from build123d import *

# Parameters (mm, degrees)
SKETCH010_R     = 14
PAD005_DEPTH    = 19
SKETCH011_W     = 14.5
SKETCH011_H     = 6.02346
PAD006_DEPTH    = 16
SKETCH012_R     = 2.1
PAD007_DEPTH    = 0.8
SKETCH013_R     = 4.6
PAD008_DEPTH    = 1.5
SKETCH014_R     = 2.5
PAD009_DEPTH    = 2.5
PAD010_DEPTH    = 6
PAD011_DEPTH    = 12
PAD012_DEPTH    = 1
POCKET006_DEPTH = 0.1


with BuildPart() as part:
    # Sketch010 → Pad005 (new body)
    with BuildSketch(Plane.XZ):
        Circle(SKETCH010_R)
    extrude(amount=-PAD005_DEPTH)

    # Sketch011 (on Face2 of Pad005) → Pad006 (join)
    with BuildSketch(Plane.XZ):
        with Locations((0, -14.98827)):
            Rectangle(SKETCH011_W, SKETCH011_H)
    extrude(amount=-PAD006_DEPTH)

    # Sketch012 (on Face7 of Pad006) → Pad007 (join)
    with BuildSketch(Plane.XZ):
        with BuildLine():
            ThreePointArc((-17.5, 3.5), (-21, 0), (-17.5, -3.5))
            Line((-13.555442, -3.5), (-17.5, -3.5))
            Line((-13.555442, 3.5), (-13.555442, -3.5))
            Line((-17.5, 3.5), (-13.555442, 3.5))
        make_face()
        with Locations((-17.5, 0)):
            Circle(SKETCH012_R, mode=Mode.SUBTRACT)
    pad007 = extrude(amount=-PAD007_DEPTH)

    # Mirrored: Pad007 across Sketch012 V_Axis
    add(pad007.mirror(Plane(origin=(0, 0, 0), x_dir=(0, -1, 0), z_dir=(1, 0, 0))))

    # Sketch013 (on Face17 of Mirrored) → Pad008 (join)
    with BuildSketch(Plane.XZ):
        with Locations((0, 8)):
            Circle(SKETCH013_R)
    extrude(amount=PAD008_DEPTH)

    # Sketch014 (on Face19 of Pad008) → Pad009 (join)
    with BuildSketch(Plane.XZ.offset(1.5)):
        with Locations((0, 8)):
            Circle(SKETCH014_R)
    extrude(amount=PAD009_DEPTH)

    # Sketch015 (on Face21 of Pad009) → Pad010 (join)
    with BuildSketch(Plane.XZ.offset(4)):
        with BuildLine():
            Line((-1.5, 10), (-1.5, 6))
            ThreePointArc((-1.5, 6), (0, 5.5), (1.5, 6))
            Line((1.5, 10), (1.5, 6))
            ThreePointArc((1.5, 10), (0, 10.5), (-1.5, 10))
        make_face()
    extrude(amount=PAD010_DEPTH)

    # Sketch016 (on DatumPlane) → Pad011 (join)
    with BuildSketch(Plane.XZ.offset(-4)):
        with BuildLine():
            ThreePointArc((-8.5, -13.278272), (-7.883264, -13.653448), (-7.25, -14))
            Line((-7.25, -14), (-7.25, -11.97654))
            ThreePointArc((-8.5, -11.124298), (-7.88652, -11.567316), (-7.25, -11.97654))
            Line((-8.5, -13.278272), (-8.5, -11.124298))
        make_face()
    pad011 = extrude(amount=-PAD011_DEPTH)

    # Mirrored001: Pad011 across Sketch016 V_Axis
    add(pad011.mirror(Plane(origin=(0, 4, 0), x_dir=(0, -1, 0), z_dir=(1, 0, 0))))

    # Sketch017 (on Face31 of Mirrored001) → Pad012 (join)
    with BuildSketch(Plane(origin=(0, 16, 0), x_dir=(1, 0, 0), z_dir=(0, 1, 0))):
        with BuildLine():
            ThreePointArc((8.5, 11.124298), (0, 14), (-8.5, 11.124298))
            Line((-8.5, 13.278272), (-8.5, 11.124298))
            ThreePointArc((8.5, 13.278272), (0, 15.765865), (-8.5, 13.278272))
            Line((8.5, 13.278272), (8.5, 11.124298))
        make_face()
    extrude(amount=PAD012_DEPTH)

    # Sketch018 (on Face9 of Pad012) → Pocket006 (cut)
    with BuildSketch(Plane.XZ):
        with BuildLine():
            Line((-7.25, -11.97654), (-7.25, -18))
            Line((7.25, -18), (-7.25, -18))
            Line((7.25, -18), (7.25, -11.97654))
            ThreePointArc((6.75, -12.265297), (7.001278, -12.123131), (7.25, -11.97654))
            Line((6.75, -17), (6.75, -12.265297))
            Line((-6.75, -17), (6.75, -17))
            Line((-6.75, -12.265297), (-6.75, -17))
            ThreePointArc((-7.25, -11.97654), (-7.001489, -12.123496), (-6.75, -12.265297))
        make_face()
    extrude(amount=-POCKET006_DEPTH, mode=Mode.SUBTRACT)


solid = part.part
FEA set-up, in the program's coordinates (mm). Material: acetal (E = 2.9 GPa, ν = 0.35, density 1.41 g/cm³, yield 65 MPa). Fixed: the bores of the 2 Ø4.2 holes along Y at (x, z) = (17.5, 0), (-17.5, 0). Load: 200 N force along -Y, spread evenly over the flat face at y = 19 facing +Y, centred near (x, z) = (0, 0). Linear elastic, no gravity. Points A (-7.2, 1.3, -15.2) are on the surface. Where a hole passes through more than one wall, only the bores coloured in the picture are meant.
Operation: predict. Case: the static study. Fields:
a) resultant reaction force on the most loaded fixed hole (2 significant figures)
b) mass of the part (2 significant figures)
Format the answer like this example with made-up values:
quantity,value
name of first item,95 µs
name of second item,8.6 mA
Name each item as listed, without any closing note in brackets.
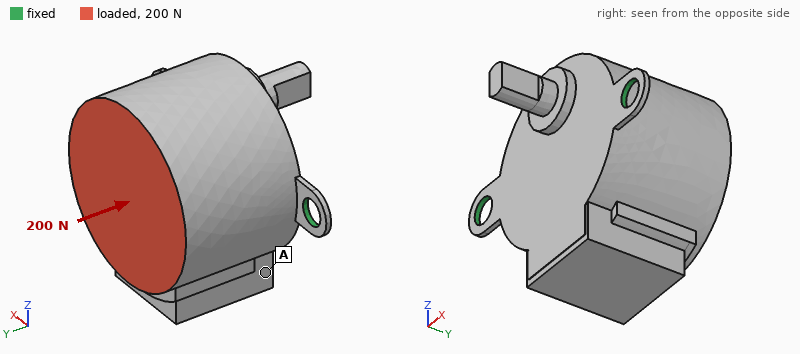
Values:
quantity,value
resultant reaction force on the most loaded fixed hole,120 N
mass of the part,19 g
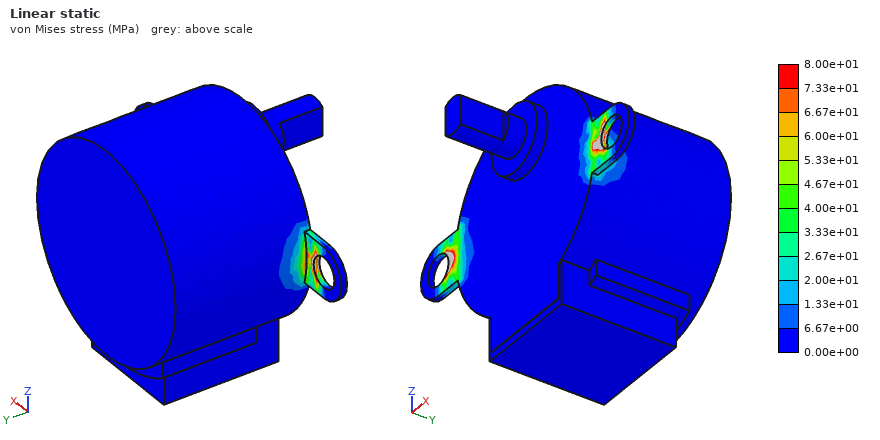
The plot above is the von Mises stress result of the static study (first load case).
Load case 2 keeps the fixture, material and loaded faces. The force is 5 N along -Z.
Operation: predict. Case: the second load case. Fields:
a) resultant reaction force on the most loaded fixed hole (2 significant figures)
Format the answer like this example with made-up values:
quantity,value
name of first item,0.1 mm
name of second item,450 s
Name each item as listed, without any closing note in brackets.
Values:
quantity,value
resultant reaction force on the most loaded fixed hole,2.5 N
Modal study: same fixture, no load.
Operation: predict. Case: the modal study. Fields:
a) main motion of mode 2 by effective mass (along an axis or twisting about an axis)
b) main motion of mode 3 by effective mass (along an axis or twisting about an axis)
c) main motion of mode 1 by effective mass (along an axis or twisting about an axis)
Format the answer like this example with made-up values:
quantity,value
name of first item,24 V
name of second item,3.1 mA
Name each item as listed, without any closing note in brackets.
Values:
quantity,value
main motion of mode 2 by effective mass,along Y
main motion of mode 3 by effective mass,along X
main motion of mode 1 by effective mass,along Z
